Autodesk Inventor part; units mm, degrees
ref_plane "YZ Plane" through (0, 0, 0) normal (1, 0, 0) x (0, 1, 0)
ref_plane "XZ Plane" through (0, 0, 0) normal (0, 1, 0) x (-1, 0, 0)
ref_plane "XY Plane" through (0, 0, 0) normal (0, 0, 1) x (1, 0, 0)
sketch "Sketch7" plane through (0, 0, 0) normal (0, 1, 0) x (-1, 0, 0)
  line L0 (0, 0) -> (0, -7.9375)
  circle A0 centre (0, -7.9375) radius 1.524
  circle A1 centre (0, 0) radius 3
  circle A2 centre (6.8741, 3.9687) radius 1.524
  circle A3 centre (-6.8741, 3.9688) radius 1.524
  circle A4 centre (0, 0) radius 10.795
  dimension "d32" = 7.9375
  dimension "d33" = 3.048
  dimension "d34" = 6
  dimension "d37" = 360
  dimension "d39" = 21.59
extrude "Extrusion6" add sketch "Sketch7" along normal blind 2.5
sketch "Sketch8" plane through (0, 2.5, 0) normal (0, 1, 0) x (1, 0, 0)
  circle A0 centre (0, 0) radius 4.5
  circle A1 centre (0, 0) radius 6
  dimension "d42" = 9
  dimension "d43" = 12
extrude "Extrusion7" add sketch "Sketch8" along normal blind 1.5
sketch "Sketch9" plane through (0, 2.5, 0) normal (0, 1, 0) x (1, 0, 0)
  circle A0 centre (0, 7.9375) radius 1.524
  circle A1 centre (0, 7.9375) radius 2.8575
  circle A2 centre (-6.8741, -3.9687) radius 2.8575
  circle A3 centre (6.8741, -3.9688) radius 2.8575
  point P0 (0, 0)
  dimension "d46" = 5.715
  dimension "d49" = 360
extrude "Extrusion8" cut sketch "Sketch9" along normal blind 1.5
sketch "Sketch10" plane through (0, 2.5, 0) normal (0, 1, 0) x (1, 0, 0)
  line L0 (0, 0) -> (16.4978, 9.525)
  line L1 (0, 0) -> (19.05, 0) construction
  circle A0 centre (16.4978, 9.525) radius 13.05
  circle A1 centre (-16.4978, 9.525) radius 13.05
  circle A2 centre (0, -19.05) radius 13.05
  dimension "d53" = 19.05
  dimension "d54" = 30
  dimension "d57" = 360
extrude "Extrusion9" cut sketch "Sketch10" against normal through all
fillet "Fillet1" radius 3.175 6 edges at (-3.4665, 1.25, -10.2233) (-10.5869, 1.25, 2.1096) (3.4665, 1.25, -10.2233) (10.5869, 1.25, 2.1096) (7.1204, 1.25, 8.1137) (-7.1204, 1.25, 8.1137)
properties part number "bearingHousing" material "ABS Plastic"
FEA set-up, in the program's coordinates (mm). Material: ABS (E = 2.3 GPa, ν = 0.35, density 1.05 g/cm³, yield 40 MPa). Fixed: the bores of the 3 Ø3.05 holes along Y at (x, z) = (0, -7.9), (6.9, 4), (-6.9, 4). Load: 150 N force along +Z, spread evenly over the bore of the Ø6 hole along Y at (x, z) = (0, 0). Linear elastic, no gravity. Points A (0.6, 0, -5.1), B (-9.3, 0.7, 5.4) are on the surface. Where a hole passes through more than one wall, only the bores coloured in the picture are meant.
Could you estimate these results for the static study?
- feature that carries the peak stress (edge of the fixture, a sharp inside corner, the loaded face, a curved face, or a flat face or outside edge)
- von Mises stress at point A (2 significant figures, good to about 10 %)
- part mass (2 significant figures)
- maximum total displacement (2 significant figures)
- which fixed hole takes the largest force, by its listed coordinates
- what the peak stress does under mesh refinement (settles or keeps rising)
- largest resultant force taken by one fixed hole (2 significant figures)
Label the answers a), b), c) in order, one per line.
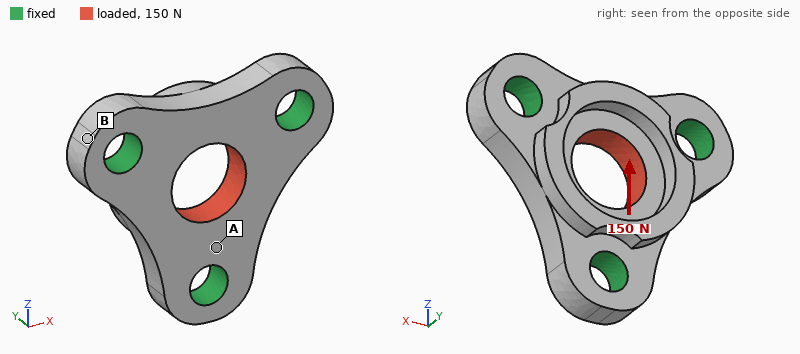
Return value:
a) edge of the fixture
b) 4.4 MPa
c) 0.51 g
d) 24 µm
e) (0, -7.9)
f) keeps rising
g) 57 N
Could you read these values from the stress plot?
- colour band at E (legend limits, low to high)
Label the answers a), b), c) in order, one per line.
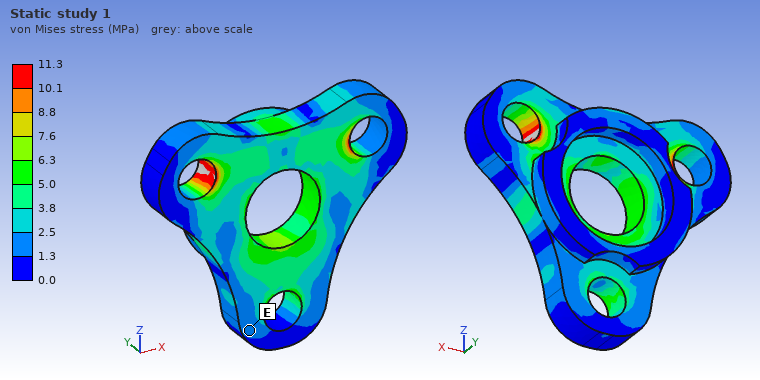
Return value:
a) 1.3 to 2.5 MPa
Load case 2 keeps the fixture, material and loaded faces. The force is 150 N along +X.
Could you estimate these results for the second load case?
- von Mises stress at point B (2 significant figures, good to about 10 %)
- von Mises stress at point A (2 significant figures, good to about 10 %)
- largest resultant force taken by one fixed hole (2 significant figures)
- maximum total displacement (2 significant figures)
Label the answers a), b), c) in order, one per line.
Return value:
a) 1.1 MPa
b) 3.9 MPa
c) 54 N
d) 21 µm
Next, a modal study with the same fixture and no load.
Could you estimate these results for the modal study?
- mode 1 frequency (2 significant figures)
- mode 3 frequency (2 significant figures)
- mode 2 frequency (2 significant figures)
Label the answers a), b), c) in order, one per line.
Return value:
a) 24 kHz
b) 24 kHz
c) 24 kHz
